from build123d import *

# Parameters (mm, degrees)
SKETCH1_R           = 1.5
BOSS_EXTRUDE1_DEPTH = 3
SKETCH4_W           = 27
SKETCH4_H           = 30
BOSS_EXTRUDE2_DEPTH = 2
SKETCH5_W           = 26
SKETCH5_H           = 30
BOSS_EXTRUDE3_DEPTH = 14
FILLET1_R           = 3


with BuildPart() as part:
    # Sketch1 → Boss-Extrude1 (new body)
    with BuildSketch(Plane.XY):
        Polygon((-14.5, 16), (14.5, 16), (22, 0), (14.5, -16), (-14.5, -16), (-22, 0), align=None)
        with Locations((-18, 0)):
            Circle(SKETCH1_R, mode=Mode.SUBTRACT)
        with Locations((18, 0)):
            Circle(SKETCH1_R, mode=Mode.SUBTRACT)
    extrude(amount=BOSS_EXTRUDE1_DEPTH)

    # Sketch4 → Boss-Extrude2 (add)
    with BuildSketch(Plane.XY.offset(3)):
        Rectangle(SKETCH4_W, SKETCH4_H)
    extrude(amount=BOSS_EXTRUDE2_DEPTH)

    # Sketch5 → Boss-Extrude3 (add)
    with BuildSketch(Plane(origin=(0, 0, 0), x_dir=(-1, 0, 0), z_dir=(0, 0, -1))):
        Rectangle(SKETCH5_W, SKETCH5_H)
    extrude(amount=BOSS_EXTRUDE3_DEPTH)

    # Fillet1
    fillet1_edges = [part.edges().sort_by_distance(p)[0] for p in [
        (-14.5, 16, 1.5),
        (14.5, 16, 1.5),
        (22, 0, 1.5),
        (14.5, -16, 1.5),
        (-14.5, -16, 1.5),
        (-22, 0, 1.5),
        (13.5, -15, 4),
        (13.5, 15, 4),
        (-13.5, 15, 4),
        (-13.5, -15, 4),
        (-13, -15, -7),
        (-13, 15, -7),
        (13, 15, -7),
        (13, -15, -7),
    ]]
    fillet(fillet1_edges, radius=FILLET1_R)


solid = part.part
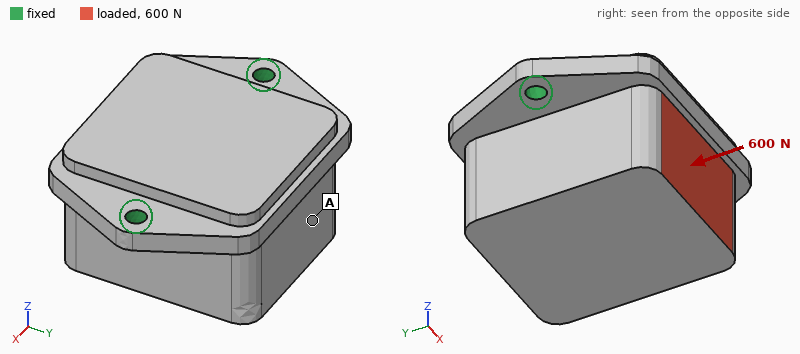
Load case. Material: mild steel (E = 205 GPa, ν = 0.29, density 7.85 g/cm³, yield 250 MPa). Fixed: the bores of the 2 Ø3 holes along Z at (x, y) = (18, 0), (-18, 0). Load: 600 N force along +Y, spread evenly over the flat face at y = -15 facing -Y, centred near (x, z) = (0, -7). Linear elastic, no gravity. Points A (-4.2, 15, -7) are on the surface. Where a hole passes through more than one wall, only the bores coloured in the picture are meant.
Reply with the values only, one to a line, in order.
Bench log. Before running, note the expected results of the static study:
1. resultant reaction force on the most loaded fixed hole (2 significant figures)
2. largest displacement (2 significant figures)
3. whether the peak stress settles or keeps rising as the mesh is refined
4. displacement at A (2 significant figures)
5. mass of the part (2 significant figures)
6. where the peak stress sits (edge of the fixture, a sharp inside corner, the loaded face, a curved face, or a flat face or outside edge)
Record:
300 N
22 µm
keeps rising
18 µm
120 g
edge of the fixture
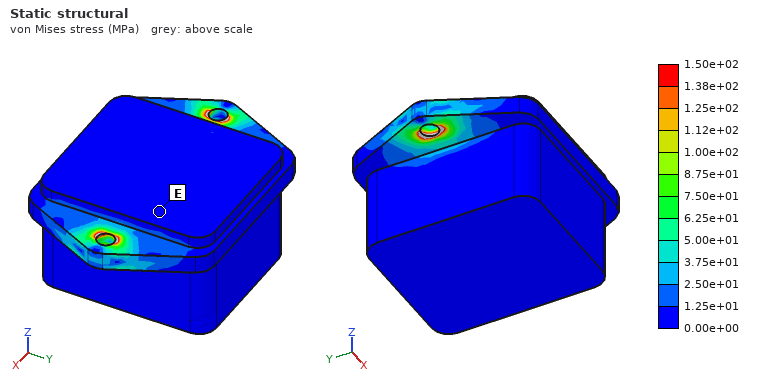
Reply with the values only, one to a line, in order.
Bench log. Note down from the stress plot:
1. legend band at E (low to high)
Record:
0.00e+00 to 1.25e+01 MPa
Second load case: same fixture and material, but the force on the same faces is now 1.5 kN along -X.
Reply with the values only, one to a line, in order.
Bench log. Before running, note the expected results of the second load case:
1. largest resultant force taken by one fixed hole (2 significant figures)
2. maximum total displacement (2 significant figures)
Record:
1.1 kN
4.9 µm
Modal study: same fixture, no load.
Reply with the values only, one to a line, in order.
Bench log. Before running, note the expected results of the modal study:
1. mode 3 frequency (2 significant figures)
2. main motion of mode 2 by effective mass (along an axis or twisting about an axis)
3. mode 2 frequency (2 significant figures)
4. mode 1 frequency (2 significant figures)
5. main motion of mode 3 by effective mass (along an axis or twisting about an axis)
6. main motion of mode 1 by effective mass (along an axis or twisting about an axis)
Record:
12 kHz
along Z
8900 Hz
2800 Hz
along X
along Y
